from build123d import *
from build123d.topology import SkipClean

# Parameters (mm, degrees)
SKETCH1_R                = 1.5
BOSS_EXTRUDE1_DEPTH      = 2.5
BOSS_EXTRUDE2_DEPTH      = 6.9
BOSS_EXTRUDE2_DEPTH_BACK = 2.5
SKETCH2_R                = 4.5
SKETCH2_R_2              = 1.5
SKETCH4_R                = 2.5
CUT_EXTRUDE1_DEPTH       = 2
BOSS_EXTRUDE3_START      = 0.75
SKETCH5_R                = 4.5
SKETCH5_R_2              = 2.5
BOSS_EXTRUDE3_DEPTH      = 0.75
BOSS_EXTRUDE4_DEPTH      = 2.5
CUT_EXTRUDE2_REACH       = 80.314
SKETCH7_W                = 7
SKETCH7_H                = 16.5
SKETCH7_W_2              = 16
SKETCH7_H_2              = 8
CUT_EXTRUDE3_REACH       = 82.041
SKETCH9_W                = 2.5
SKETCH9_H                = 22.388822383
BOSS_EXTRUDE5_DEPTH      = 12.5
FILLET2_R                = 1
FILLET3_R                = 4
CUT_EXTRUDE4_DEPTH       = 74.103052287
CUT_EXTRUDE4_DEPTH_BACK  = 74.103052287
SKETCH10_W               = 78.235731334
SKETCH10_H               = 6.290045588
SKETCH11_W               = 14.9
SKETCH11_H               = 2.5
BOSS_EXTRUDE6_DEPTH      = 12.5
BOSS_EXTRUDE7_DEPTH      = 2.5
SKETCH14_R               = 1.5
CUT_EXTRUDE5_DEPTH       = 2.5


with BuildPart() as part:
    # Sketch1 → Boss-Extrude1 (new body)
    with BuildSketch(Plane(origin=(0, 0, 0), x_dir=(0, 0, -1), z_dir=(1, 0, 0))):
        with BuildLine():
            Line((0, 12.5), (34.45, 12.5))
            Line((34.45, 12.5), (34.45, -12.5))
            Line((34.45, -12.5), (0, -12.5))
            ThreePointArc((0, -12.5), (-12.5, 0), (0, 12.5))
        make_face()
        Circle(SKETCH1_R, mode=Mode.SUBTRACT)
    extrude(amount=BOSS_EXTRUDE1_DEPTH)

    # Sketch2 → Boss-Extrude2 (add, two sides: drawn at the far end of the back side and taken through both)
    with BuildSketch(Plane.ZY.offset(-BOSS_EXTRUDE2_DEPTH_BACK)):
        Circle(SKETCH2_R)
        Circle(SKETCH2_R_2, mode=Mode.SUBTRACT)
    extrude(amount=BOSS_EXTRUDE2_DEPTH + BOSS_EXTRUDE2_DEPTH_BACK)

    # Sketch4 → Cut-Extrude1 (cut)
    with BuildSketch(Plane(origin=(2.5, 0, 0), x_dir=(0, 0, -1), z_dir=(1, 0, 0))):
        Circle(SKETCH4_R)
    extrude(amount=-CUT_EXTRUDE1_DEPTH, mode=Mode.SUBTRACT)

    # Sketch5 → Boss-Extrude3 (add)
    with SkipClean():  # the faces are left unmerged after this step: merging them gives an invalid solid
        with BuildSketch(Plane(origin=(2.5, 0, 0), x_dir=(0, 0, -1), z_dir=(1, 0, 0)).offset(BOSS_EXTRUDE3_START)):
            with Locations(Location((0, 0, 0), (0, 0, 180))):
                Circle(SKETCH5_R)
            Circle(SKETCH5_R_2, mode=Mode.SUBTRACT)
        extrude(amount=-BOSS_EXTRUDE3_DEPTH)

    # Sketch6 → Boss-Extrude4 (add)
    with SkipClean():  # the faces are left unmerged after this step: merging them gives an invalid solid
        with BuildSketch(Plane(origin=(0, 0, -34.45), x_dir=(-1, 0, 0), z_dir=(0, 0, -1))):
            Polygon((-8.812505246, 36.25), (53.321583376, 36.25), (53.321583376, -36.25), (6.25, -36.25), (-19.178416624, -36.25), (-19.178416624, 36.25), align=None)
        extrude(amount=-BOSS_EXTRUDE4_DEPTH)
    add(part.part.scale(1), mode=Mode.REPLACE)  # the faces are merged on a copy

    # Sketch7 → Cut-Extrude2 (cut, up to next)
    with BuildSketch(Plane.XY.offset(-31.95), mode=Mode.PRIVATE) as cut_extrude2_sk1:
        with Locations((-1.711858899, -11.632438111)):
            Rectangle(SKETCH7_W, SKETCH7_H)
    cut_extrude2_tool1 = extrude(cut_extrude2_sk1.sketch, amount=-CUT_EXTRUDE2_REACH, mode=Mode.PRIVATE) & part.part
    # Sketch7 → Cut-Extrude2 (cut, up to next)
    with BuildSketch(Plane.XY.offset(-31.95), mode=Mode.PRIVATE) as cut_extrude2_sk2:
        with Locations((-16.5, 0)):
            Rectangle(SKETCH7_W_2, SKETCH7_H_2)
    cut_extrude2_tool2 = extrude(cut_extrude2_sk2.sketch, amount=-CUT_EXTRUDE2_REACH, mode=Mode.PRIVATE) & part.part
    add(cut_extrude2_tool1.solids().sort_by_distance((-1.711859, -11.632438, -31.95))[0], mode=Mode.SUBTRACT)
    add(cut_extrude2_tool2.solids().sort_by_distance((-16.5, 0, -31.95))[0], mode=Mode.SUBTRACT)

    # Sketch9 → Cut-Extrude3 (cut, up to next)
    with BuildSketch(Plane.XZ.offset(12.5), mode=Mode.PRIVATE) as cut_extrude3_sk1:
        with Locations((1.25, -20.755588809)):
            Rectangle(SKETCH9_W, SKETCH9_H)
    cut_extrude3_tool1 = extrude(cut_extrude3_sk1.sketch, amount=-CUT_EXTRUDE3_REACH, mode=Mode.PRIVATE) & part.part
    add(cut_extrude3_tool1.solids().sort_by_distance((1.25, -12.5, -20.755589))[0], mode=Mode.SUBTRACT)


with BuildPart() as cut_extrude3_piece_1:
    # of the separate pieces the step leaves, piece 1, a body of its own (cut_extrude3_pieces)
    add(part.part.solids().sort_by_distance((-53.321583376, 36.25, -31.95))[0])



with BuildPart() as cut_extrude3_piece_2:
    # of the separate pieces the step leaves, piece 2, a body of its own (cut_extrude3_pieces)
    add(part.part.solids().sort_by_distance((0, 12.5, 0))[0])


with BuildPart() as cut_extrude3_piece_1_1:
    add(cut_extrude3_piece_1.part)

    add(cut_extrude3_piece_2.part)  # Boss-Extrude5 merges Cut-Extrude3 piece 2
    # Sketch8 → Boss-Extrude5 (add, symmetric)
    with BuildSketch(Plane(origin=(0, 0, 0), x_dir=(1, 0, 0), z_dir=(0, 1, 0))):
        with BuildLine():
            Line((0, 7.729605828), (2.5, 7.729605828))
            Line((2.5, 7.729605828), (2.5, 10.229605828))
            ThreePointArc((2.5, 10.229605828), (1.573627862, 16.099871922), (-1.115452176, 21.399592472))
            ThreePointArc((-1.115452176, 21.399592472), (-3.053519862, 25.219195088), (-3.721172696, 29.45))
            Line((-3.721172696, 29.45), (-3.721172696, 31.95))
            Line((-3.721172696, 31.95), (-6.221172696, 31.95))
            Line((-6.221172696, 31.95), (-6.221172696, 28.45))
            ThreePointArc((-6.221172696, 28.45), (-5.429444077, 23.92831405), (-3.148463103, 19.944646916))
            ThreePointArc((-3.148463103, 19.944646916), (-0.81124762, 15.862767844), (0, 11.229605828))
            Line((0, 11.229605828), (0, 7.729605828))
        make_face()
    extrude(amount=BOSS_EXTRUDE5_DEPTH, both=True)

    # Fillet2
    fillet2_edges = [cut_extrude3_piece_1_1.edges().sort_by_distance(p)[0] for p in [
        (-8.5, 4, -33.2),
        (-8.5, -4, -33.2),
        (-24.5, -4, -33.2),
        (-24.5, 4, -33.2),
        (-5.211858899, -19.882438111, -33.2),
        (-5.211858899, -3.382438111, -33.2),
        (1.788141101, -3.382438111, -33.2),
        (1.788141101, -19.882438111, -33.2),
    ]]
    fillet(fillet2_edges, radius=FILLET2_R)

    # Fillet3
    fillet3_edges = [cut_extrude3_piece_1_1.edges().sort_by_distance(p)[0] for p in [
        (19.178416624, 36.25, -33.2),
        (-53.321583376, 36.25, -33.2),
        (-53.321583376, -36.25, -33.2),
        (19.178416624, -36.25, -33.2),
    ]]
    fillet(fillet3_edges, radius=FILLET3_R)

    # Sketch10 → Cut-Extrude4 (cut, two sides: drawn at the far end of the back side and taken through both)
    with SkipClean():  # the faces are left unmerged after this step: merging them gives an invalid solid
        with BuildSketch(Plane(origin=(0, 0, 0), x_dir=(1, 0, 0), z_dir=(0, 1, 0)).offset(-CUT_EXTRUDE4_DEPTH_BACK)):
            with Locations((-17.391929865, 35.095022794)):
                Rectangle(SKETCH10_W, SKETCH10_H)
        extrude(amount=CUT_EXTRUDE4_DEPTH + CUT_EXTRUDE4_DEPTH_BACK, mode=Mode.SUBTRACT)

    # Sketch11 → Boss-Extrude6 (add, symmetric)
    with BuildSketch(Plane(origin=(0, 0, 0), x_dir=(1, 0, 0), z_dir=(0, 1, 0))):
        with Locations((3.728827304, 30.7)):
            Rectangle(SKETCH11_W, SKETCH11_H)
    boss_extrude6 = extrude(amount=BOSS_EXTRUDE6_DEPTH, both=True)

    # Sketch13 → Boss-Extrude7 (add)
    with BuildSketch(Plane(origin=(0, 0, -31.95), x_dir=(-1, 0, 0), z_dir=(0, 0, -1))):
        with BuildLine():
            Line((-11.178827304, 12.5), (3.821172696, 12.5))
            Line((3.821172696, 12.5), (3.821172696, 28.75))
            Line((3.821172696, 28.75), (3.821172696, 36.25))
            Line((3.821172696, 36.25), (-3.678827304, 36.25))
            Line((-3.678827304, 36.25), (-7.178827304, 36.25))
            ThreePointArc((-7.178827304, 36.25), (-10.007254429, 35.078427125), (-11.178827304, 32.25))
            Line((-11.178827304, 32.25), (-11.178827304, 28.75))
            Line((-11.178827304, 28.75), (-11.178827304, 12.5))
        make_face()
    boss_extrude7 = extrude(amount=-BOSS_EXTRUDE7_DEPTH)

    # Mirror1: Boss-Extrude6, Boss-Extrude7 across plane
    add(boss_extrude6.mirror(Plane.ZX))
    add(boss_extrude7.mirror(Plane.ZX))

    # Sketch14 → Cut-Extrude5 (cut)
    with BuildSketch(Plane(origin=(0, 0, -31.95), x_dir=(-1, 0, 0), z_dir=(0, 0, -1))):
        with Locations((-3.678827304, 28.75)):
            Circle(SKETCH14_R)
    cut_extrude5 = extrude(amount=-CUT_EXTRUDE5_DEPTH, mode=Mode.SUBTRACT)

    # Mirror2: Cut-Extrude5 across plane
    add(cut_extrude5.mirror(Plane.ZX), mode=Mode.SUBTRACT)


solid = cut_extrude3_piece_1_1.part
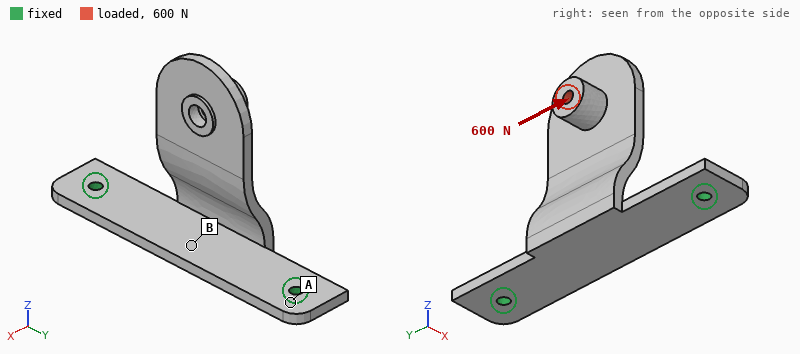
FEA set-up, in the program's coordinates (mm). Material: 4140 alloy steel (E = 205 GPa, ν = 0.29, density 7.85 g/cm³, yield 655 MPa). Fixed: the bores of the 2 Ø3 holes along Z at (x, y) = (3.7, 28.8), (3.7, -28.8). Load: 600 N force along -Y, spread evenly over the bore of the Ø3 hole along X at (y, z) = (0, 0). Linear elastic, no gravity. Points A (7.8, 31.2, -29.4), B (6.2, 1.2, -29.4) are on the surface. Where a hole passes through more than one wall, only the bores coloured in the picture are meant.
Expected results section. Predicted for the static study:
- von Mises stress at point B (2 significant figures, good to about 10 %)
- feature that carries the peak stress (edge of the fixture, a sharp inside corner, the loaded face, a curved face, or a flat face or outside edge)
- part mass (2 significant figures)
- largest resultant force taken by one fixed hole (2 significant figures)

100 MPa
a curved face
45 g
550 N
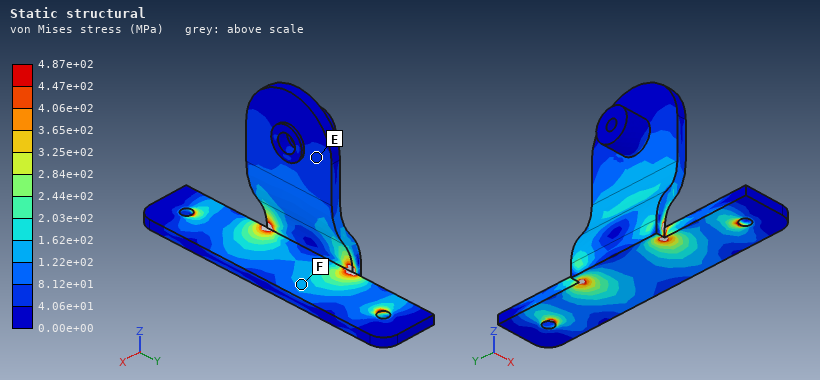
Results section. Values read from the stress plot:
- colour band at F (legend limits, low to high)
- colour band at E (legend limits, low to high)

1.22e+02 to 1.62e+02 MPa
4.06e+01 to 8.12e+01 MPa
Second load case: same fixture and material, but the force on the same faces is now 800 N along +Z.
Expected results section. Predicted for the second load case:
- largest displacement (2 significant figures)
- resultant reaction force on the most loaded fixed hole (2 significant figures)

0.55 mm
410 N
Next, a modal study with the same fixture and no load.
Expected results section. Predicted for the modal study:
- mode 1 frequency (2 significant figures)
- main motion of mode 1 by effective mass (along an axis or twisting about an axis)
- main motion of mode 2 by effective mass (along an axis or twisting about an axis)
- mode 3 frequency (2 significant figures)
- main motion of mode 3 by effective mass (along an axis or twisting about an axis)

700 Hz
along X
along Y
2400 Hz
along Z
